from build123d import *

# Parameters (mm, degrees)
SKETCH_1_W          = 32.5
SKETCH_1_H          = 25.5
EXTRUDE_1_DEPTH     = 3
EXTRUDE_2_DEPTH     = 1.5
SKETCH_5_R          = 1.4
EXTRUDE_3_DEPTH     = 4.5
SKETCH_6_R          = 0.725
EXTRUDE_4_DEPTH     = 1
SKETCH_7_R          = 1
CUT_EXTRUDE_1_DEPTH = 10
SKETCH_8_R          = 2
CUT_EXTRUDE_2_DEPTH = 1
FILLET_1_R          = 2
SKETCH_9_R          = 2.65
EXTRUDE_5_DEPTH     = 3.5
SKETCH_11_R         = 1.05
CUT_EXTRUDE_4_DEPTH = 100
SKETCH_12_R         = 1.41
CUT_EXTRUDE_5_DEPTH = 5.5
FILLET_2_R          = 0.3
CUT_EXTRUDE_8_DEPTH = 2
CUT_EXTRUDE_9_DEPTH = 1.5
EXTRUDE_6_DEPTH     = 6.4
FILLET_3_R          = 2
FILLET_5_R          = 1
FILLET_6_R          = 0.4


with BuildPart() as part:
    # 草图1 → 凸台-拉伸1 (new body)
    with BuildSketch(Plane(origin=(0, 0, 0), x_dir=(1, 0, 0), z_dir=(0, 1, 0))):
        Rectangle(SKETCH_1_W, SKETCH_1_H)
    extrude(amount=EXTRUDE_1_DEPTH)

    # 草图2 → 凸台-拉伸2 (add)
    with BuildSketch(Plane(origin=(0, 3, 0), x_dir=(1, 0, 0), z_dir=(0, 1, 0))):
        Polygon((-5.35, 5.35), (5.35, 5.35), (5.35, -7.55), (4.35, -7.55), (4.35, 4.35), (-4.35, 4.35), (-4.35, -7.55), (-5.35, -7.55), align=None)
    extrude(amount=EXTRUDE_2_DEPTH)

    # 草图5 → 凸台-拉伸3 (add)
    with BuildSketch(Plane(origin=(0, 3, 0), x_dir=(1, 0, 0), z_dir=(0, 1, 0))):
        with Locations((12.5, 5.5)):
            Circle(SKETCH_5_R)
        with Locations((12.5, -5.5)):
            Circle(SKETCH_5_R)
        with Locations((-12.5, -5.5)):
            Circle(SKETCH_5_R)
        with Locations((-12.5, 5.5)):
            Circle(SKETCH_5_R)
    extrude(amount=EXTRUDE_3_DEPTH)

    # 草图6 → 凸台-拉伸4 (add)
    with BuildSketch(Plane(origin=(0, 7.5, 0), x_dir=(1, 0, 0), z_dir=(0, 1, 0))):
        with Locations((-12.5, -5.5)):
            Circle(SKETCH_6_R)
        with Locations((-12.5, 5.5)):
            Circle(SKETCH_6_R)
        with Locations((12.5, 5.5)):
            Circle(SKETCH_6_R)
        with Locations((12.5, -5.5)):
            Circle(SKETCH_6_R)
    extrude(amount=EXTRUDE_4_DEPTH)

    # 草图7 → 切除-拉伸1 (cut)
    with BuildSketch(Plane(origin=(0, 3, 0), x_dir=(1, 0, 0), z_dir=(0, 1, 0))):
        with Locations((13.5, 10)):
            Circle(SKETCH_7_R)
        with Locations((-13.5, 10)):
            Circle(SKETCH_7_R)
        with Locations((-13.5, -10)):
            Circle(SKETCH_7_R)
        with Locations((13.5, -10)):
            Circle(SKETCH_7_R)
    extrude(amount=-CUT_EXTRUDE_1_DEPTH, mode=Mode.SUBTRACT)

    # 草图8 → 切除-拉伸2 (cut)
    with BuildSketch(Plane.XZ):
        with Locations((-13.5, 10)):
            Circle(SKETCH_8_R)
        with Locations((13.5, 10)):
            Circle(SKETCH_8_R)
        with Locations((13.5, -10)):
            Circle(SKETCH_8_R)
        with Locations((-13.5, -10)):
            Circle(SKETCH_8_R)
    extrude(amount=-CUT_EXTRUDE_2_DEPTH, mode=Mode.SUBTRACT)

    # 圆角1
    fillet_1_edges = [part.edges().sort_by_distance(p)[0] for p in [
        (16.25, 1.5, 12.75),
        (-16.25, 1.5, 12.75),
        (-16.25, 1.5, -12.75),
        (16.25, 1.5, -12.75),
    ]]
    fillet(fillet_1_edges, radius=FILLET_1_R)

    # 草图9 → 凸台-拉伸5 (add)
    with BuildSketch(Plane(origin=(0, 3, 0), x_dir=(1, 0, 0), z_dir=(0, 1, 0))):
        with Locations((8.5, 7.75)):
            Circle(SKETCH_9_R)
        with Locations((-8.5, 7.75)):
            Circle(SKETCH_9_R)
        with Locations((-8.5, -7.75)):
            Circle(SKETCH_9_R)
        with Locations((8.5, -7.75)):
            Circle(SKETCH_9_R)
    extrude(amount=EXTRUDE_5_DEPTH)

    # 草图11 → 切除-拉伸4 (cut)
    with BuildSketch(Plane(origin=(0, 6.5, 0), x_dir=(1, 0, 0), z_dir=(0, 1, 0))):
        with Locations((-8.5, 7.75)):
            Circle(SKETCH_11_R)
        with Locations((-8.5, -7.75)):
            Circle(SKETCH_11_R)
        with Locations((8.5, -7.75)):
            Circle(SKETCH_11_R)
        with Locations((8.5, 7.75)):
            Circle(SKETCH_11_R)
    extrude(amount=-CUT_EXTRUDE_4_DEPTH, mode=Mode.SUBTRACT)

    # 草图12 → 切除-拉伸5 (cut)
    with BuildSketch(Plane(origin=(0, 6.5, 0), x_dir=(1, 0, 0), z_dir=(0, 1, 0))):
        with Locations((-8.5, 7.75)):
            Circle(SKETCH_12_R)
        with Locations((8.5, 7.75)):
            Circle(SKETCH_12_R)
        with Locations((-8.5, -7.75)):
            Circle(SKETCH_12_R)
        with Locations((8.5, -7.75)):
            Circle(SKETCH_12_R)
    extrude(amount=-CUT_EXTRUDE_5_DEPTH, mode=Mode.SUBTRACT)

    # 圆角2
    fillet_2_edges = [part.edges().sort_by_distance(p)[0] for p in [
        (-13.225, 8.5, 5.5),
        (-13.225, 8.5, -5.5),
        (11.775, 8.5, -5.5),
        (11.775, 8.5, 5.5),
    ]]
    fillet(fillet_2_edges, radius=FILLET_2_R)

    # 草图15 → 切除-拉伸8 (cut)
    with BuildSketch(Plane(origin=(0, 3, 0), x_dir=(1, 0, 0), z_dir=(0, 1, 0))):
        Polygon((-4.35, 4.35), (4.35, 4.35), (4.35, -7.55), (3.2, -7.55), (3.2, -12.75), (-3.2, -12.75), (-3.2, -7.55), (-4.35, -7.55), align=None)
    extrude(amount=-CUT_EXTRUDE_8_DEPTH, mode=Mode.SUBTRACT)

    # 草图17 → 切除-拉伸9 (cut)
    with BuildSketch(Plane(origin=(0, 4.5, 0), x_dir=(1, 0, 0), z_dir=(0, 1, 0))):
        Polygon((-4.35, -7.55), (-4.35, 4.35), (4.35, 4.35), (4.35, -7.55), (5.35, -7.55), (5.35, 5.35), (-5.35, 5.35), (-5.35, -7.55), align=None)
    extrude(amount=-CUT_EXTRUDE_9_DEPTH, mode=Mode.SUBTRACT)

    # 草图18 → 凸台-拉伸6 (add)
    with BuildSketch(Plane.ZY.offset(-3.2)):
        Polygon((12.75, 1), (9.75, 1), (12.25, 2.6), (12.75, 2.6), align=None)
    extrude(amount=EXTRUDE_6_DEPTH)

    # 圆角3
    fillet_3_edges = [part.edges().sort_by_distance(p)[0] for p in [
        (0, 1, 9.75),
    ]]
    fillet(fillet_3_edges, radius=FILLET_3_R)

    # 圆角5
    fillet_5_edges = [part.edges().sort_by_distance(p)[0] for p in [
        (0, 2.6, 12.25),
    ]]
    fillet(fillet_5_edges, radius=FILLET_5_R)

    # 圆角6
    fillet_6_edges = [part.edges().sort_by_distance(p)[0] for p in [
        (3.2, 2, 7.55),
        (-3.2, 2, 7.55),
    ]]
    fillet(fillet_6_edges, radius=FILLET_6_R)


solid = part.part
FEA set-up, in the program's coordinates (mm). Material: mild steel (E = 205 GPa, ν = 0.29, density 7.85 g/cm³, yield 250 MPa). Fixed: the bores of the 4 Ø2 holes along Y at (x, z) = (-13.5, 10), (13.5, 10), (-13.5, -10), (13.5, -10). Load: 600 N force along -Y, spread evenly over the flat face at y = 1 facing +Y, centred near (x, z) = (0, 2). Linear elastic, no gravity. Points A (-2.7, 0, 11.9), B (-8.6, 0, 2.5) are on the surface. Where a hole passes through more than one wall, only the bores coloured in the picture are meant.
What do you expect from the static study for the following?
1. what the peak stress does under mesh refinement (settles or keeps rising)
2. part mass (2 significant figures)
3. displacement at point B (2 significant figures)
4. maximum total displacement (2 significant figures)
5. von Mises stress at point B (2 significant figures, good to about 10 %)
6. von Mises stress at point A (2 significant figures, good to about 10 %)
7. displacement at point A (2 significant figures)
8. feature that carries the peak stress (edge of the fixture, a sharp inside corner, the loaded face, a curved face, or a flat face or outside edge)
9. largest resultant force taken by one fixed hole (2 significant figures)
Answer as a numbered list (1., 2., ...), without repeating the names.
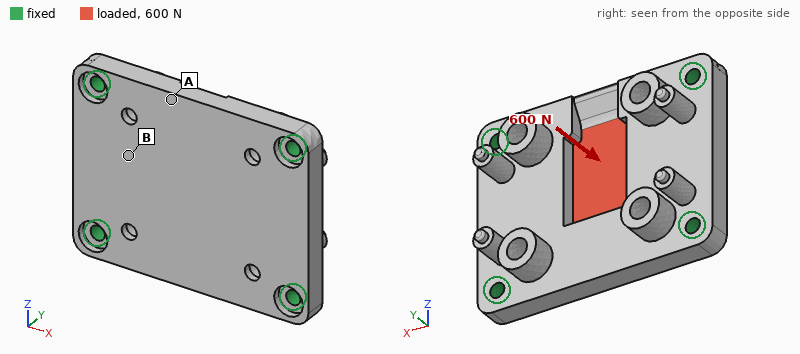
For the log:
1. keeps rising
2. 19 g
3. 8.0 µm
4. 22 µm
5. 31 MPa
6. 66 MPa
7. 12 µm
8. edge of the fixture
9. 470 N
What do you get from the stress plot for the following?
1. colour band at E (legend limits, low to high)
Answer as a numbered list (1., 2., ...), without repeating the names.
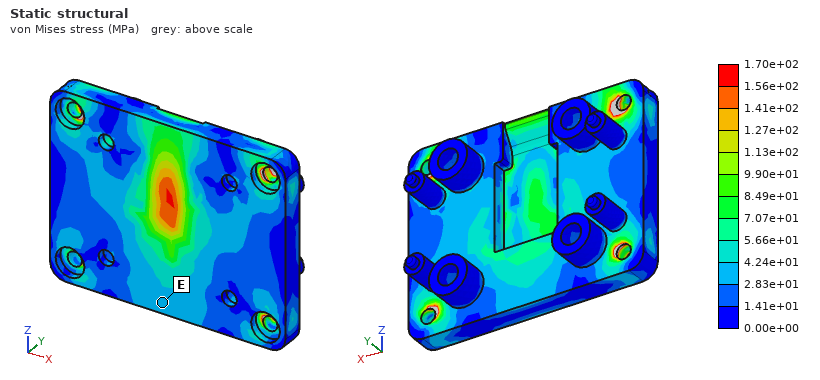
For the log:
1. 2.83e+01 to 4.24e+01 MPa
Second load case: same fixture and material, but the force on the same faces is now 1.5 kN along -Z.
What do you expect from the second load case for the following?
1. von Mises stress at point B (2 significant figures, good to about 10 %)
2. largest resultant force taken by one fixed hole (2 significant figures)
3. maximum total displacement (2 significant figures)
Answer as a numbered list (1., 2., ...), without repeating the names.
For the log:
1. 22 MPa
2. 450 N
3. 3.7 µm
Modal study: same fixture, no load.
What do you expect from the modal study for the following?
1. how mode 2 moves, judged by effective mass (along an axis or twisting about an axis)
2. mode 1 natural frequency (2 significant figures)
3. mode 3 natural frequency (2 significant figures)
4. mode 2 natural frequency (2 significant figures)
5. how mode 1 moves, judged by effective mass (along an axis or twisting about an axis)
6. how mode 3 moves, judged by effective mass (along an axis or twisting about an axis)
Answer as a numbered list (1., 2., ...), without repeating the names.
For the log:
1. twisting about X
2. 14 kHz
3. 25 kHz
4. 21 kHz
5. along Y
6. twisting about Z
